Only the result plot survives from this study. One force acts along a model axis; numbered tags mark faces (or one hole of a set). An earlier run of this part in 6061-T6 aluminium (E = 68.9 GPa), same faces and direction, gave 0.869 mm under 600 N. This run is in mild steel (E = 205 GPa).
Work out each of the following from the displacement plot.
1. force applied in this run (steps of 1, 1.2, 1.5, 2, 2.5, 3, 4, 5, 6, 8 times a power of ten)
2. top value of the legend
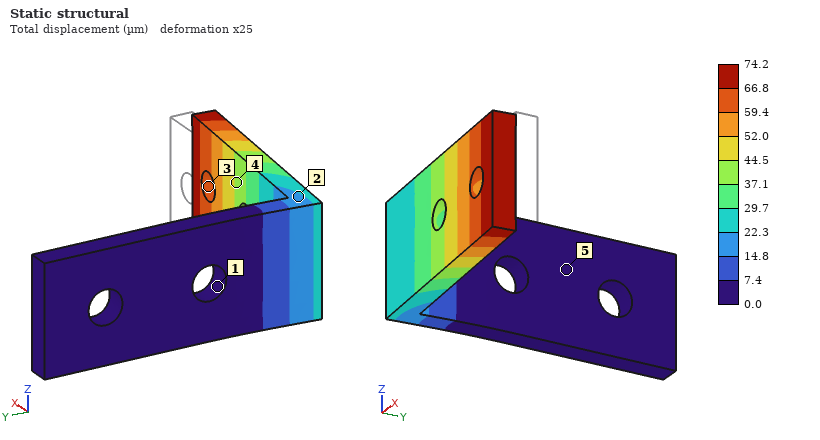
150 N
74.2 µm
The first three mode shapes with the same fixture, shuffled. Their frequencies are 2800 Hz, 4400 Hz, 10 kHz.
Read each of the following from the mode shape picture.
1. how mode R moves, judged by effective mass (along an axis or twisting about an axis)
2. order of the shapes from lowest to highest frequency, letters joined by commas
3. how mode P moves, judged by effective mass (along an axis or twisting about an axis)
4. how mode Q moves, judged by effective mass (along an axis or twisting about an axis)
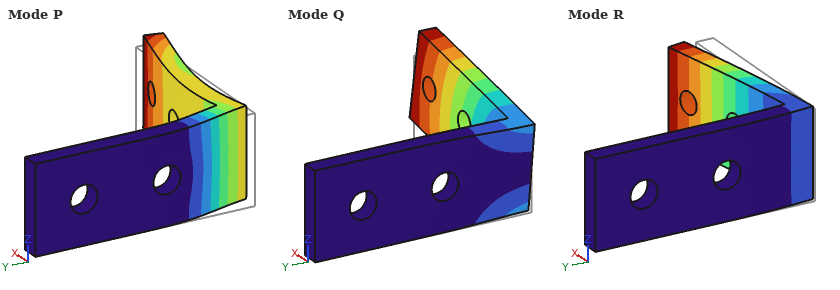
along Y
R, Q, P
along X
along Z
